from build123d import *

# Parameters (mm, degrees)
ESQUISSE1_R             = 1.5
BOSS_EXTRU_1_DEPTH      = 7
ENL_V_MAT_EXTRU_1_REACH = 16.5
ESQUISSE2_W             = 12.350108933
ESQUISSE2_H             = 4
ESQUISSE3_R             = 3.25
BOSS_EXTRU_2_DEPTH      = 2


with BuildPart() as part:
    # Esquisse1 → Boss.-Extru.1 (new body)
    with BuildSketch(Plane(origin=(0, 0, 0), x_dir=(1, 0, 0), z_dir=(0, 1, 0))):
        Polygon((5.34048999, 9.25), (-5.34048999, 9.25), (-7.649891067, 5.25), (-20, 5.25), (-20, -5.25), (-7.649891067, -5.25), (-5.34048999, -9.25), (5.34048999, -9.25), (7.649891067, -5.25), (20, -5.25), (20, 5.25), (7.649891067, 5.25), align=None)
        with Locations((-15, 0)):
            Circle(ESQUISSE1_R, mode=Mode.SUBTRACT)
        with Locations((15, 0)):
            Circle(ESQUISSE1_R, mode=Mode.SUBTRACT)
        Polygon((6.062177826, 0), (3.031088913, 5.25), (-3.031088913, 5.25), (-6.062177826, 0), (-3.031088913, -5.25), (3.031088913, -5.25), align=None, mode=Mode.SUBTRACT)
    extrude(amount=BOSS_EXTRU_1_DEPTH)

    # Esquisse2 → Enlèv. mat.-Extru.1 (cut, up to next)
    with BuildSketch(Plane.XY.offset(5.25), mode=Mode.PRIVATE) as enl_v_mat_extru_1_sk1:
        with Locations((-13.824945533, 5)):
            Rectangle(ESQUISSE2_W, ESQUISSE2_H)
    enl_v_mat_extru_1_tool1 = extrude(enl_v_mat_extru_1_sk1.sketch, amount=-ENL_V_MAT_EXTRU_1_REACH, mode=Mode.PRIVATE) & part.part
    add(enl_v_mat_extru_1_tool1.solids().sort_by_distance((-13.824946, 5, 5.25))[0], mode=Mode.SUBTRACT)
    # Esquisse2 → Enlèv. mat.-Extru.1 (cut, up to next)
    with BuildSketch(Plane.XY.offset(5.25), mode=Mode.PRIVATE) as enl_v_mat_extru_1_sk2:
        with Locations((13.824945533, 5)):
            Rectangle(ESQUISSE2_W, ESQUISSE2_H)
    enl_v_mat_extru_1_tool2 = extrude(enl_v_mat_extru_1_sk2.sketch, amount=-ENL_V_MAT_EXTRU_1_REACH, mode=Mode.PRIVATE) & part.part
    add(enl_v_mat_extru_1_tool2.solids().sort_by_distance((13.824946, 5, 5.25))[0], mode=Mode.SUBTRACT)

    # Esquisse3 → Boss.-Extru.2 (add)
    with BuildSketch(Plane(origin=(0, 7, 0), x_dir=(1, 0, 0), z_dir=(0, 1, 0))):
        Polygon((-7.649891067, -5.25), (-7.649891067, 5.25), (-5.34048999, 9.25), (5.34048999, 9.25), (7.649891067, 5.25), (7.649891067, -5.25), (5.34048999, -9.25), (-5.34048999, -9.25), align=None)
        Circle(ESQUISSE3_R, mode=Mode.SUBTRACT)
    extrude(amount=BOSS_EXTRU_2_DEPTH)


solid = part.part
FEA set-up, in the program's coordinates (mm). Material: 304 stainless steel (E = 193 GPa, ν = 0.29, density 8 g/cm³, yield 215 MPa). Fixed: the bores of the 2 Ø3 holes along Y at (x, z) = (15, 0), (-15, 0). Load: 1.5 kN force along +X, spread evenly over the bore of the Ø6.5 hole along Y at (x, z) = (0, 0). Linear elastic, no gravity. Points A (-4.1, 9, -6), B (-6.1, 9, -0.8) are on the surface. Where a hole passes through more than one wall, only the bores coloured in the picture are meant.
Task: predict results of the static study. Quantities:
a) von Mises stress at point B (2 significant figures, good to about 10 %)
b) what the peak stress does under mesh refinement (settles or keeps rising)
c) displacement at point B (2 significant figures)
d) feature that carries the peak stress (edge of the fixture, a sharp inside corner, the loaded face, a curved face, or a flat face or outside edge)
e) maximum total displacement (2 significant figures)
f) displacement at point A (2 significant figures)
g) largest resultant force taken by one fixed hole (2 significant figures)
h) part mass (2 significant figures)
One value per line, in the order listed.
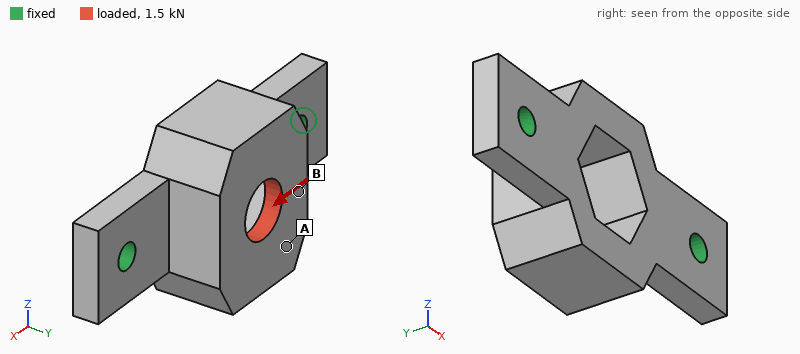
40 MPa
keeps rising
8.6 µm
edge of the fixture
9.3 µm
7.2 µm
870 N
19 g
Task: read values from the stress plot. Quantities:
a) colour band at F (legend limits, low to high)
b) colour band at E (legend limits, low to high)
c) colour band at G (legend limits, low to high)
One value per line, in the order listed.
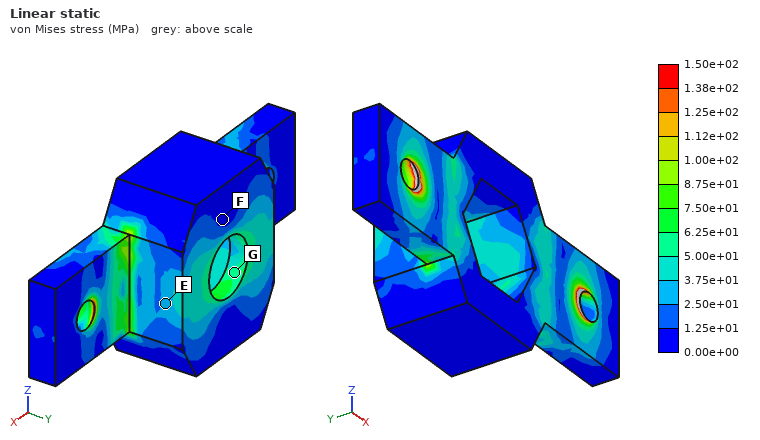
0.00e+00 to 1.25e+01 MPa
2.50e+01 to 3.75e+01 MPa
5.00e+01 to 6.25e+01 MPa
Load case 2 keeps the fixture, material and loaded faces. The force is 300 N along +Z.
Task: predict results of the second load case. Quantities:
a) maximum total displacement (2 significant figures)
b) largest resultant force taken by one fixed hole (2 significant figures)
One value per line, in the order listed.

14 µm
150 N
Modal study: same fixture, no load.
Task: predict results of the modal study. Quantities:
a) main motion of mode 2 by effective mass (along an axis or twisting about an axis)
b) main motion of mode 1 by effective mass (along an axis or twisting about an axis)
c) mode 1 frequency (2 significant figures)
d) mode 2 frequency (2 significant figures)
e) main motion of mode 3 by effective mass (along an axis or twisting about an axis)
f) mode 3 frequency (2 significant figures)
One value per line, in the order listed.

along Y
along Z
8000 Hz
14 kHz
along X
24 kHz
